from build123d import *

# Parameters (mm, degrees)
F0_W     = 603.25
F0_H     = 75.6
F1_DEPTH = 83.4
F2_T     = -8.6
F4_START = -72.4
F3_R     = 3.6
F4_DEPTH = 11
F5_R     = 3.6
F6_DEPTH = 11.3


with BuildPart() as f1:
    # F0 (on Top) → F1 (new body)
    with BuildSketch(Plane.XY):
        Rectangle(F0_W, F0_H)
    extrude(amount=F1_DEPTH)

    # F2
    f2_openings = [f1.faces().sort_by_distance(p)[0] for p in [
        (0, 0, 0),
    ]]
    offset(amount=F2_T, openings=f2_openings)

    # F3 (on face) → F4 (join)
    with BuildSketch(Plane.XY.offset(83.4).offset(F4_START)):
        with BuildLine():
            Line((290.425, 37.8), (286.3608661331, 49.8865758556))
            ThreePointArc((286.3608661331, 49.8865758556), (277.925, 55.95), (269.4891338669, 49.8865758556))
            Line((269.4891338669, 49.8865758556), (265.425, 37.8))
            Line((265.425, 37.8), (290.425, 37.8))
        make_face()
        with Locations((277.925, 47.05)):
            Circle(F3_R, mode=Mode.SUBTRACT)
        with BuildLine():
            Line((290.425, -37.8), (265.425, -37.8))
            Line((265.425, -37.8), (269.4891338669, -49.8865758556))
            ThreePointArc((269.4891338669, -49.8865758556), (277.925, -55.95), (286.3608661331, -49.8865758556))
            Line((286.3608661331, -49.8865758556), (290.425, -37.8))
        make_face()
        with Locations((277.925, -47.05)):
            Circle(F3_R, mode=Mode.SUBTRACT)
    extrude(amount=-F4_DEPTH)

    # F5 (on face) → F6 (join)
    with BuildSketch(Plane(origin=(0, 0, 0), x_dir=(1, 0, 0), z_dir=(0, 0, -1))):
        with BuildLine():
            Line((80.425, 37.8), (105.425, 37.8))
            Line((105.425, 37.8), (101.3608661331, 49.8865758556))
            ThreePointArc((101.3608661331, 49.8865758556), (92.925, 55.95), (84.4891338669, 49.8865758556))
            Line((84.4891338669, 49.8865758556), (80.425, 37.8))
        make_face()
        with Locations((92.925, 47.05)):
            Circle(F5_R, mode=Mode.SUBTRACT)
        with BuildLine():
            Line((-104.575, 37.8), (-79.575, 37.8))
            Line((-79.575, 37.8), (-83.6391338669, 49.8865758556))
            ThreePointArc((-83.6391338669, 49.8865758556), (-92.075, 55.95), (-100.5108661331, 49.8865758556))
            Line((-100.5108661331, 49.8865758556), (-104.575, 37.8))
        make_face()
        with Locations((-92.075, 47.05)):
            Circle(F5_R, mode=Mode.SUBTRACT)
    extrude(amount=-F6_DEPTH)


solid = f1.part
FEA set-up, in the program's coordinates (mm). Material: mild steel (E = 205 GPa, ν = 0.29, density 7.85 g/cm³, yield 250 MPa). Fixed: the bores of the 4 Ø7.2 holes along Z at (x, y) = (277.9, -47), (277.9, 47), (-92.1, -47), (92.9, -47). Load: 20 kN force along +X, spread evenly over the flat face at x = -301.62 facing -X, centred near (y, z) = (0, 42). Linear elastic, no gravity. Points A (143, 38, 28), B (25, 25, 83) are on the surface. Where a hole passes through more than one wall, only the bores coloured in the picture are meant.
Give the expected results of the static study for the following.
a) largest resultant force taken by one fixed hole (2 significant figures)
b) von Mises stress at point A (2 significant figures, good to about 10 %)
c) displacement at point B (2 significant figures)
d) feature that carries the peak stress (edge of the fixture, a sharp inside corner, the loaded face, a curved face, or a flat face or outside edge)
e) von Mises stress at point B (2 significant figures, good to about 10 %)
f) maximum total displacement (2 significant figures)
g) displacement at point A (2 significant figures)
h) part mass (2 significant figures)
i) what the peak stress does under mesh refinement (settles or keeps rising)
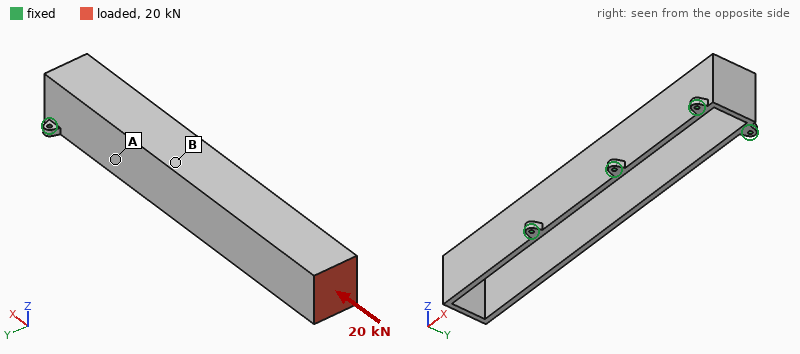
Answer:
6.8 kN
13 MPa
0.032 mm
edge of the fixture
6.5 MPa
0.12 mm
0.025 mm
9.9 kg
keeps rising
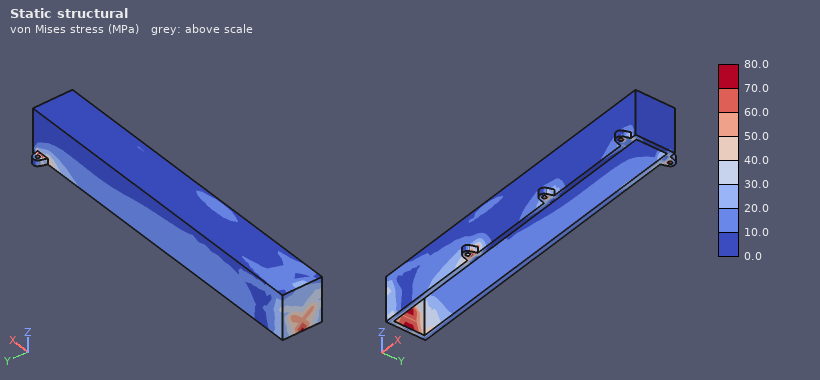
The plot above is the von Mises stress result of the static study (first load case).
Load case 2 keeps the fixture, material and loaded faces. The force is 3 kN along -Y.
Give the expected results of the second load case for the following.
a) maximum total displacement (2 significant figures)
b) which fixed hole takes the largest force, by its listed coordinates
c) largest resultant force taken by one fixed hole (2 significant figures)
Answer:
0.63 mm
(277.9, 47)
6.0 kN
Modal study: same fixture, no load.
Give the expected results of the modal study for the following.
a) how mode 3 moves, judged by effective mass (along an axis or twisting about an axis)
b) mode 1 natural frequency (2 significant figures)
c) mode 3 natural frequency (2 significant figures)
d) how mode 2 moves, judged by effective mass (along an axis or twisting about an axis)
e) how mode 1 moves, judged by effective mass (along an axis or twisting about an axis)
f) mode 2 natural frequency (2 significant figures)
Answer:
along Y
280 Hz
600 Hz
along Z
along Y
330 Hz
